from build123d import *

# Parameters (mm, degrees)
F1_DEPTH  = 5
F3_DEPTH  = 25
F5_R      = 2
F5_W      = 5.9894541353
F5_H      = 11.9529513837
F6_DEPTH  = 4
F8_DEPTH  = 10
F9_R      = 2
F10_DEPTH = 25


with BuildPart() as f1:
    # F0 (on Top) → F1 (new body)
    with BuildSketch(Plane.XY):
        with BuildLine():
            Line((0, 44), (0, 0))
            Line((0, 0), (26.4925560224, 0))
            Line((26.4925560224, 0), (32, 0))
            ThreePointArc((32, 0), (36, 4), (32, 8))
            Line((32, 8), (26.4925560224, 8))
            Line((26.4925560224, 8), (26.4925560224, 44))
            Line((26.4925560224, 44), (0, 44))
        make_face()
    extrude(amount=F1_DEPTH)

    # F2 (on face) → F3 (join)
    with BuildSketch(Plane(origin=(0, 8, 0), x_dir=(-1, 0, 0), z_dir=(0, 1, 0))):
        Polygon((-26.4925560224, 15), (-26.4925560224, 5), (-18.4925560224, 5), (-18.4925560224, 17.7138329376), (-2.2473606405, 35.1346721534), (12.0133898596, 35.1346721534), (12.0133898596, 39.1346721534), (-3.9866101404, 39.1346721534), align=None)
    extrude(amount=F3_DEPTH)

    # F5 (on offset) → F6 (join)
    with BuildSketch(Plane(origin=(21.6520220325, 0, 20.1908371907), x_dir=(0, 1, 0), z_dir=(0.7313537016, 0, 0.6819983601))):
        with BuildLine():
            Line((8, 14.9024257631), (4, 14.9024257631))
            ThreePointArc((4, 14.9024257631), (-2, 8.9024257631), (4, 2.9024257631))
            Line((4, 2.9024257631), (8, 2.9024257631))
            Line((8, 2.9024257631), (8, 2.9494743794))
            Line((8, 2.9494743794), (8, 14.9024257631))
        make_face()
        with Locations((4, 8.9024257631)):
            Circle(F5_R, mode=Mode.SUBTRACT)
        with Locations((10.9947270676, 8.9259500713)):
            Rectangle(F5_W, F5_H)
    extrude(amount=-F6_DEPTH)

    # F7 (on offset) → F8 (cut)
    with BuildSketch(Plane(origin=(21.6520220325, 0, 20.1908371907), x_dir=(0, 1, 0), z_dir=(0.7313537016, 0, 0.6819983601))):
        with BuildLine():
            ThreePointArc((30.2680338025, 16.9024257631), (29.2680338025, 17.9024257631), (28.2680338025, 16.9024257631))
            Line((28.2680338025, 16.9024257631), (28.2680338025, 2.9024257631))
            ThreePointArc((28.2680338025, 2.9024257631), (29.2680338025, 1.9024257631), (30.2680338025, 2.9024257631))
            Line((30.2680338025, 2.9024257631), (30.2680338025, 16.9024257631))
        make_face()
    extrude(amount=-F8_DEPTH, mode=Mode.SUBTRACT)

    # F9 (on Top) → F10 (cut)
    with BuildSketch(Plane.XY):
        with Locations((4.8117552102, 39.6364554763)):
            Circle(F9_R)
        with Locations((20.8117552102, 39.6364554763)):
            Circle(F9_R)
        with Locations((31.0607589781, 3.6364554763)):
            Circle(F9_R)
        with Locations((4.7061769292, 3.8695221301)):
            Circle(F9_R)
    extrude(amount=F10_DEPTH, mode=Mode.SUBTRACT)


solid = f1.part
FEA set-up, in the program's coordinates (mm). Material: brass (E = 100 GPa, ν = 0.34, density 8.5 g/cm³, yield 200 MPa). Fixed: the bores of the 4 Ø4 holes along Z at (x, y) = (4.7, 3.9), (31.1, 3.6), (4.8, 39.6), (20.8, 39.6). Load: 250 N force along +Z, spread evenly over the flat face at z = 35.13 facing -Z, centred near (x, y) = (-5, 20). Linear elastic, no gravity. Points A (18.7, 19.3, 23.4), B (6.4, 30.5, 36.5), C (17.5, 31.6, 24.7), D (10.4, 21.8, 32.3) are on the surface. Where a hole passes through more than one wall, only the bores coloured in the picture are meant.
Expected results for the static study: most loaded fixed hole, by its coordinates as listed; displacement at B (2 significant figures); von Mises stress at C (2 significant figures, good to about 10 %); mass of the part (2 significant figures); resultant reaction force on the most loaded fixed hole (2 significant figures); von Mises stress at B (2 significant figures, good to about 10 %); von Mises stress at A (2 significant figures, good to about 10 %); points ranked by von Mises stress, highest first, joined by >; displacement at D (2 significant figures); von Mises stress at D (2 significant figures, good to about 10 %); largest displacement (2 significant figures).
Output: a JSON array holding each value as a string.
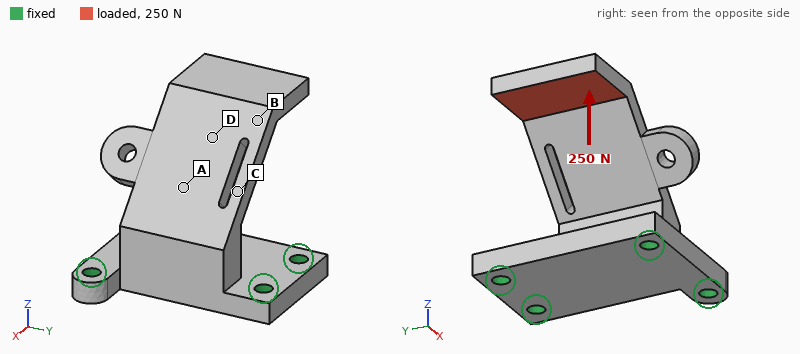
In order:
["(4.7, 3.9)", "0.16 mm", "88 MPa", "110 g", "220 N", "29 MPa", "72 MPa", "C > A > D > B", "0.11 mm", "47 MPa", "0.33 mm"]
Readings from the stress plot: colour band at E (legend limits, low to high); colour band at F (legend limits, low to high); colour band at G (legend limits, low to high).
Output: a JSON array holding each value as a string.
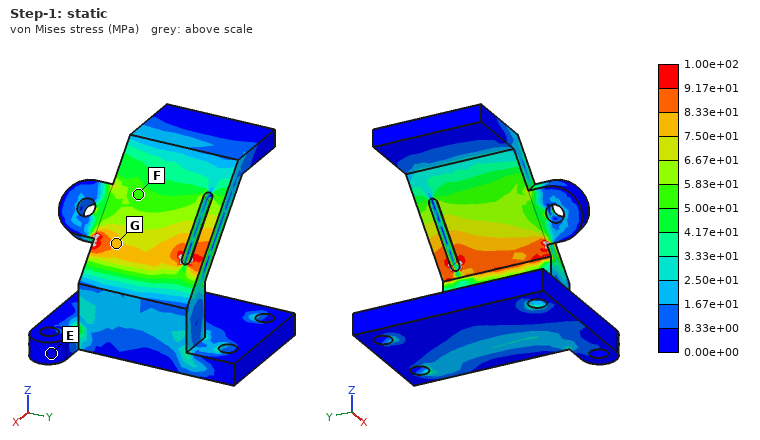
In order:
["0.00e+00 to 8.33e+00 MPa", "5.00e+01 to 5.83e+01 MPa", "7.50e+01 to 8.33e+01 MPa"]
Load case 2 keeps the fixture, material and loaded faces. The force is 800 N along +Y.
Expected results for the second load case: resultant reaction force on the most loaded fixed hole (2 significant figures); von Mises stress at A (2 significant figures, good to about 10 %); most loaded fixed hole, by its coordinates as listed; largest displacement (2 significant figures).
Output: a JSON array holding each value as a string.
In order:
["1.1 kN", "50 MPa", "(20.8, 39.6)", "0.28 mm"]
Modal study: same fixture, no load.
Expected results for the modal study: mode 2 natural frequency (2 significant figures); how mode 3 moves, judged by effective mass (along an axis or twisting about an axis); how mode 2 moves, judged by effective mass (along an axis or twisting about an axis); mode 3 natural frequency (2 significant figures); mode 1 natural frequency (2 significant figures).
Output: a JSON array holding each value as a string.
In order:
["2500 Hz", "along X", "along Y", "3800 Hz", "1100 Hz"]
